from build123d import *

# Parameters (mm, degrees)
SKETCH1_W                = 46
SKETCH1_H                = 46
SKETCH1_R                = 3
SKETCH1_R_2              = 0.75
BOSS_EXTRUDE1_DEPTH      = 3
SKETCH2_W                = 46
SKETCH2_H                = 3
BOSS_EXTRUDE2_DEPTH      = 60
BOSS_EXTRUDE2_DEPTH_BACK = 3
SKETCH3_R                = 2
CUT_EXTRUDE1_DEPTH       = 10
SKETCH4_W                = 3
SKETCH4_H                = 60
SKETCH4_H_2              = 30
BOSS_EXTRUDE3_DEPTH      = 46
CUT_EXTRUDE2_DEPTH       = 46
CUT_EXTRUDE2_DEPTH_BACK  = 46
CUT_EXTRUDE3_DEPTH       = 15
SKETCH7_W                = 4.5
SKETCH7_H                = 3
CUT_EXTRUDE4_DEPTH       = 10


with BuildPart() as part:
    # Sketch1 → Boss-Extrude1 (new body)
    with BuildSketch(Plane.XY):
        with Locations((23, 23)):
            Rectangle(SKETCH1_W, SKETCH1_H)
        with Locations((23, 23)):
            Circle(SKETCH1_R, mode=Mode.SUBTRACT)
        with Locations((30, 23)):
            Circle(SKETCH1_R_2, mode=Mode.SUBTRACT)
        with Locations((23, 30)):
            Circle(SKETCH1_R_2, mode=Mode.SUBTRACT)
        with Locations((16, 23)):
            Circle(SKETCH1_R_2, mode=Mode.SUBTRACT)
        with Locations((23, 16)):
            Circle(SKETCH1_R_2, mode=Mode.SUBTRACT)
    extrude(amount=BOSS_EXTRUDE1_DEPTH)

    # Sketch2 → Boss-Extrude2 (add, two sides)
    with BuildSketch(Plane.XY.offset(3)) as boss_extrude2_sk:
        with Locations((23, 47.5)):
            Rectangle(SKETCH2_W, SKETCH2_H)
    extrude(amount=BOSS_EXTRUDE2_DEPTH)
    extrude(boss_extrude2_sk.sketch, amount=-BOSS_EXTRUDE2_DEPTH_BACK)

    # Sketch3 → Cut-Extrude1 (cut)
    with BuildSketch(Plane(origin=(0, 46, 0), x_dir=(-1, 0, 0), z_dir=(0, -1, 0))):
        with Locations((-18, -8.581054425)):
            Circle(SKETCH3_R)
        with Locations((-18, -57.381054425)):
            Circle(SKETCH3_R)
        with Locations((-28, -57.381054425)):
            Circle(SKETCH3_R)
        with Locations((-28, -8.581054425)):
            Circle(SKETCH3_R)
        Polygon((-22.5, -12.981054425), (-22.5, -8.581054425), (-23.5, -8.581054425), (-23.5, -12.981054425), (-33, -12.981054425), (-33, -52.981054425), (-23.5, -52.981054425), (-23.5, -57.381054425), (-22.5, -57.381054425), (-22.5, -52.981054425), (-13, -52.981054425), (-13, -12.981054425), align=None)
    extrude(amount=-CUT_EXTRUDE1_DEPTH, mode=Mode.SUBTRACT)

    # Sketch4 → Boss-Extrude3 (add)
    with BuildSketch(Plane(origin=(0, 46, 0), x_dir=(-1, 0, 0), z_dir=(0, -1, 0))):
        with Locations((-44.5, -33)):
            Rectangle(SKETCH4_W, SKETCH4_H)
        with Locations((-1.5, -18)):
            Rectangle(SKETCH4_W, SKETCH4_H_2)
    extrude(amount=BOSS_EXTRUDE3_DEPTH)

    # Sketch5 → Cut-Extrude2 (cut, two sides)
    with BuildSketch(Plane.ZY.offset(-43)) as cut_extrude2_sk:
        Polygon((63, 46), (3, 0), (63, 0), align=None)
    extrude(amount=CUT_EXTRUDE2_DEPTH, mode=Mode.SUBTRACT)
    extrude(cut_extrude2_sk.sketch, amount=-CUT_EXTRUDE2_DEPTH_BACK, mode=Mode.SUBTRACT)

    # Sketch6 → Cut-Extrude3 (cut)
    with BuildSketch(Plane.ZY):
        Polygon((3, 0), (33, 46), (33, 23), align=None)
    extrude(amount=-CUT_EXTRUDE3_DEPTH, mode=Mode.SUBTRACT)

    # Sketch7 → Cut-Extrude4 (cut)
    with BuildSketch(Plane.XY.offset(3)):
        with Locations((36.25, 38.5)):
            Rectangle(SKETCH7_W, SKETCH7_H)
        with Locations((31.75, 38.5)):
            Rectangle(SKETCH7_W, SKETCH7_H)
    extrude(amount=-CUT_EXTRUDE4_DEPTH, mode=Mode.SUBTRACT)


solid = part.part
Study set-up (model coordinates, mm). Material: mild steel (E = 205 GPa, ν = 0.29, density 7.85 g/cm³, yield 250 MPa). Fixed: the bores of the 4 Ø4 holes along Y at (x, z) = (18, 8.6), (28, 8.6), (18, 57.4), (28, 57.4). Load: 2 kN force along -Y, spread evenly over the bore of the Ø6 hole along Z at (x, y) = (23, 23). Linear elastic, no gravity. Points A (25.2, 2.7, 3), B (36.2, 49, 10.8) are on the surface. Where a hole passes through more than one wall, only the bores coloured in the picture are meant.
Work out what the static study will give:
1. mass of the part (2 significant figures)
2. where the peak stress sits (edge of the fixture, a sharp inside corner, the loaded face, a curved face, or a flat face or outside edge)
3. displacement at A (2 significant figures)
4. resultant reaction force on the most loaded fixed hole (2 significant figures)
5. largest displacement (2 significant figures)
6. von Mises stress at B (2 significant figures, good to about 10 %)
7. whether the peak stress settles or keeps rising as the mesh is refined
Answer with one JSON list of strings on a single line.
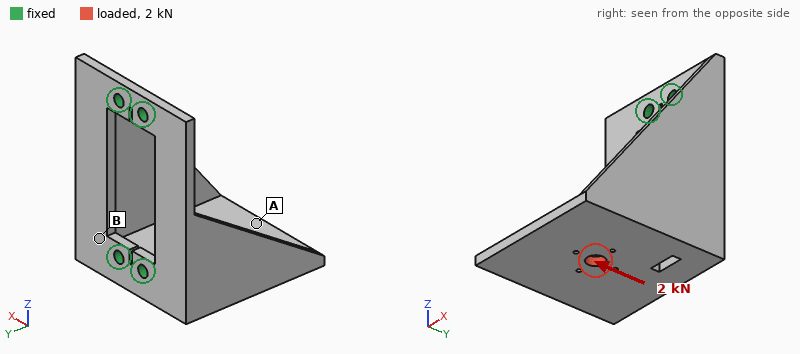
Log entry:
["150 g", "edge of the fixture", "30 µm", "1.1 kN", "39 µm", "25 MPa", "keeps rising"]
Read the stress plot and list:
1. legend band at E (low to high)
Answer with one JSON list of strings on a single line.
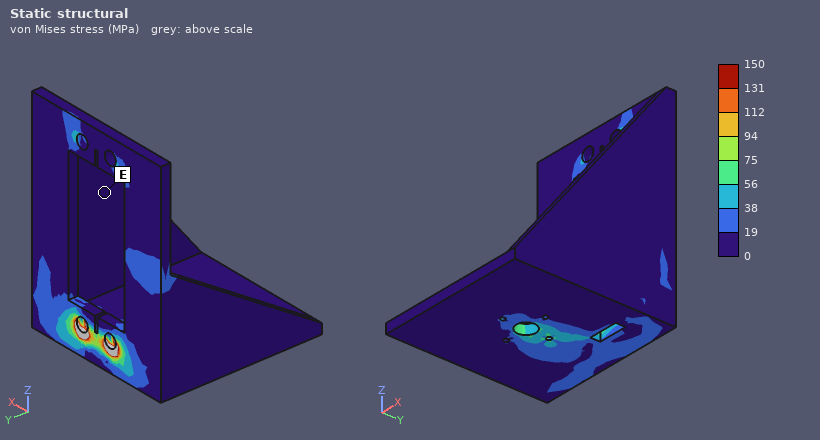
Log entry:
["0 to 19 MPa"]
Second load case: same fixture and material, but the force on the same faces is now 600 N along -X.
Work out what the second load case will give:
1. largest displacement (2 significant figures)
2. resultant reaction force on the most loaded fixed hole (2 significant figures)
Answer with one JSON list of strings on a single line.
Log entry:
["68 µm", "960 N"]
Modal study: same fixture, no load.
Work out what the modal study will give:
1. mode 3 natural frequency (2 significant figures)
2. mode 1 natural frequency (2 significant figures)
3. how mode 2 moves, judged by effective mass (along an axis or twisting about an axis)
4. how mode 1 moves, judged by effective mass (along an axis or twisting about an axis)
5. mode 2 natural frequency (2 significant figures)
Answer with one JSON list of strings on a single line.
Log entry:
["3200 Hz", "1800 Hz", "along Z", "along X", "2100 Hz"]
